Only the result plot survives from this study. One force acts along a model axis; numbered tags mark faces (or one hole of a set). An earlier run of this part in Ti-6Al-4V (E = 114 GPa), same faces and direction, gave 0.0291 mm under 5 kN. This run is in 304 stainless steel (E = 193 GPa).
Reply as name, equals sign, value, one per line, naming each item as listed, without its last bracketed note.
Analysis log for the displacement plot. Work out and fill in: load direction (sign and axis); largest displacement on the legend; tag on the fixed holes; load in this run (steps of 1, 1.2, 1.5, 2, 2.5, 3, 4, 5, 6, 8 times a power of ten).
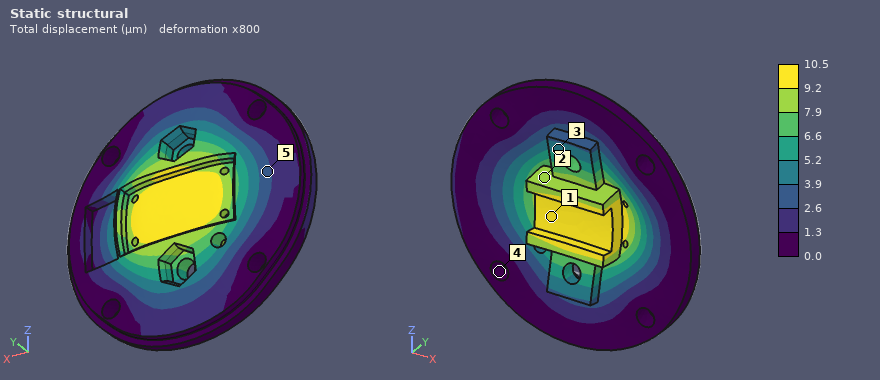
load direction = +Y
largest displacement on the legend = 10.5 µm
tag on the fixed holes = 4
load in this run = 3 kN
